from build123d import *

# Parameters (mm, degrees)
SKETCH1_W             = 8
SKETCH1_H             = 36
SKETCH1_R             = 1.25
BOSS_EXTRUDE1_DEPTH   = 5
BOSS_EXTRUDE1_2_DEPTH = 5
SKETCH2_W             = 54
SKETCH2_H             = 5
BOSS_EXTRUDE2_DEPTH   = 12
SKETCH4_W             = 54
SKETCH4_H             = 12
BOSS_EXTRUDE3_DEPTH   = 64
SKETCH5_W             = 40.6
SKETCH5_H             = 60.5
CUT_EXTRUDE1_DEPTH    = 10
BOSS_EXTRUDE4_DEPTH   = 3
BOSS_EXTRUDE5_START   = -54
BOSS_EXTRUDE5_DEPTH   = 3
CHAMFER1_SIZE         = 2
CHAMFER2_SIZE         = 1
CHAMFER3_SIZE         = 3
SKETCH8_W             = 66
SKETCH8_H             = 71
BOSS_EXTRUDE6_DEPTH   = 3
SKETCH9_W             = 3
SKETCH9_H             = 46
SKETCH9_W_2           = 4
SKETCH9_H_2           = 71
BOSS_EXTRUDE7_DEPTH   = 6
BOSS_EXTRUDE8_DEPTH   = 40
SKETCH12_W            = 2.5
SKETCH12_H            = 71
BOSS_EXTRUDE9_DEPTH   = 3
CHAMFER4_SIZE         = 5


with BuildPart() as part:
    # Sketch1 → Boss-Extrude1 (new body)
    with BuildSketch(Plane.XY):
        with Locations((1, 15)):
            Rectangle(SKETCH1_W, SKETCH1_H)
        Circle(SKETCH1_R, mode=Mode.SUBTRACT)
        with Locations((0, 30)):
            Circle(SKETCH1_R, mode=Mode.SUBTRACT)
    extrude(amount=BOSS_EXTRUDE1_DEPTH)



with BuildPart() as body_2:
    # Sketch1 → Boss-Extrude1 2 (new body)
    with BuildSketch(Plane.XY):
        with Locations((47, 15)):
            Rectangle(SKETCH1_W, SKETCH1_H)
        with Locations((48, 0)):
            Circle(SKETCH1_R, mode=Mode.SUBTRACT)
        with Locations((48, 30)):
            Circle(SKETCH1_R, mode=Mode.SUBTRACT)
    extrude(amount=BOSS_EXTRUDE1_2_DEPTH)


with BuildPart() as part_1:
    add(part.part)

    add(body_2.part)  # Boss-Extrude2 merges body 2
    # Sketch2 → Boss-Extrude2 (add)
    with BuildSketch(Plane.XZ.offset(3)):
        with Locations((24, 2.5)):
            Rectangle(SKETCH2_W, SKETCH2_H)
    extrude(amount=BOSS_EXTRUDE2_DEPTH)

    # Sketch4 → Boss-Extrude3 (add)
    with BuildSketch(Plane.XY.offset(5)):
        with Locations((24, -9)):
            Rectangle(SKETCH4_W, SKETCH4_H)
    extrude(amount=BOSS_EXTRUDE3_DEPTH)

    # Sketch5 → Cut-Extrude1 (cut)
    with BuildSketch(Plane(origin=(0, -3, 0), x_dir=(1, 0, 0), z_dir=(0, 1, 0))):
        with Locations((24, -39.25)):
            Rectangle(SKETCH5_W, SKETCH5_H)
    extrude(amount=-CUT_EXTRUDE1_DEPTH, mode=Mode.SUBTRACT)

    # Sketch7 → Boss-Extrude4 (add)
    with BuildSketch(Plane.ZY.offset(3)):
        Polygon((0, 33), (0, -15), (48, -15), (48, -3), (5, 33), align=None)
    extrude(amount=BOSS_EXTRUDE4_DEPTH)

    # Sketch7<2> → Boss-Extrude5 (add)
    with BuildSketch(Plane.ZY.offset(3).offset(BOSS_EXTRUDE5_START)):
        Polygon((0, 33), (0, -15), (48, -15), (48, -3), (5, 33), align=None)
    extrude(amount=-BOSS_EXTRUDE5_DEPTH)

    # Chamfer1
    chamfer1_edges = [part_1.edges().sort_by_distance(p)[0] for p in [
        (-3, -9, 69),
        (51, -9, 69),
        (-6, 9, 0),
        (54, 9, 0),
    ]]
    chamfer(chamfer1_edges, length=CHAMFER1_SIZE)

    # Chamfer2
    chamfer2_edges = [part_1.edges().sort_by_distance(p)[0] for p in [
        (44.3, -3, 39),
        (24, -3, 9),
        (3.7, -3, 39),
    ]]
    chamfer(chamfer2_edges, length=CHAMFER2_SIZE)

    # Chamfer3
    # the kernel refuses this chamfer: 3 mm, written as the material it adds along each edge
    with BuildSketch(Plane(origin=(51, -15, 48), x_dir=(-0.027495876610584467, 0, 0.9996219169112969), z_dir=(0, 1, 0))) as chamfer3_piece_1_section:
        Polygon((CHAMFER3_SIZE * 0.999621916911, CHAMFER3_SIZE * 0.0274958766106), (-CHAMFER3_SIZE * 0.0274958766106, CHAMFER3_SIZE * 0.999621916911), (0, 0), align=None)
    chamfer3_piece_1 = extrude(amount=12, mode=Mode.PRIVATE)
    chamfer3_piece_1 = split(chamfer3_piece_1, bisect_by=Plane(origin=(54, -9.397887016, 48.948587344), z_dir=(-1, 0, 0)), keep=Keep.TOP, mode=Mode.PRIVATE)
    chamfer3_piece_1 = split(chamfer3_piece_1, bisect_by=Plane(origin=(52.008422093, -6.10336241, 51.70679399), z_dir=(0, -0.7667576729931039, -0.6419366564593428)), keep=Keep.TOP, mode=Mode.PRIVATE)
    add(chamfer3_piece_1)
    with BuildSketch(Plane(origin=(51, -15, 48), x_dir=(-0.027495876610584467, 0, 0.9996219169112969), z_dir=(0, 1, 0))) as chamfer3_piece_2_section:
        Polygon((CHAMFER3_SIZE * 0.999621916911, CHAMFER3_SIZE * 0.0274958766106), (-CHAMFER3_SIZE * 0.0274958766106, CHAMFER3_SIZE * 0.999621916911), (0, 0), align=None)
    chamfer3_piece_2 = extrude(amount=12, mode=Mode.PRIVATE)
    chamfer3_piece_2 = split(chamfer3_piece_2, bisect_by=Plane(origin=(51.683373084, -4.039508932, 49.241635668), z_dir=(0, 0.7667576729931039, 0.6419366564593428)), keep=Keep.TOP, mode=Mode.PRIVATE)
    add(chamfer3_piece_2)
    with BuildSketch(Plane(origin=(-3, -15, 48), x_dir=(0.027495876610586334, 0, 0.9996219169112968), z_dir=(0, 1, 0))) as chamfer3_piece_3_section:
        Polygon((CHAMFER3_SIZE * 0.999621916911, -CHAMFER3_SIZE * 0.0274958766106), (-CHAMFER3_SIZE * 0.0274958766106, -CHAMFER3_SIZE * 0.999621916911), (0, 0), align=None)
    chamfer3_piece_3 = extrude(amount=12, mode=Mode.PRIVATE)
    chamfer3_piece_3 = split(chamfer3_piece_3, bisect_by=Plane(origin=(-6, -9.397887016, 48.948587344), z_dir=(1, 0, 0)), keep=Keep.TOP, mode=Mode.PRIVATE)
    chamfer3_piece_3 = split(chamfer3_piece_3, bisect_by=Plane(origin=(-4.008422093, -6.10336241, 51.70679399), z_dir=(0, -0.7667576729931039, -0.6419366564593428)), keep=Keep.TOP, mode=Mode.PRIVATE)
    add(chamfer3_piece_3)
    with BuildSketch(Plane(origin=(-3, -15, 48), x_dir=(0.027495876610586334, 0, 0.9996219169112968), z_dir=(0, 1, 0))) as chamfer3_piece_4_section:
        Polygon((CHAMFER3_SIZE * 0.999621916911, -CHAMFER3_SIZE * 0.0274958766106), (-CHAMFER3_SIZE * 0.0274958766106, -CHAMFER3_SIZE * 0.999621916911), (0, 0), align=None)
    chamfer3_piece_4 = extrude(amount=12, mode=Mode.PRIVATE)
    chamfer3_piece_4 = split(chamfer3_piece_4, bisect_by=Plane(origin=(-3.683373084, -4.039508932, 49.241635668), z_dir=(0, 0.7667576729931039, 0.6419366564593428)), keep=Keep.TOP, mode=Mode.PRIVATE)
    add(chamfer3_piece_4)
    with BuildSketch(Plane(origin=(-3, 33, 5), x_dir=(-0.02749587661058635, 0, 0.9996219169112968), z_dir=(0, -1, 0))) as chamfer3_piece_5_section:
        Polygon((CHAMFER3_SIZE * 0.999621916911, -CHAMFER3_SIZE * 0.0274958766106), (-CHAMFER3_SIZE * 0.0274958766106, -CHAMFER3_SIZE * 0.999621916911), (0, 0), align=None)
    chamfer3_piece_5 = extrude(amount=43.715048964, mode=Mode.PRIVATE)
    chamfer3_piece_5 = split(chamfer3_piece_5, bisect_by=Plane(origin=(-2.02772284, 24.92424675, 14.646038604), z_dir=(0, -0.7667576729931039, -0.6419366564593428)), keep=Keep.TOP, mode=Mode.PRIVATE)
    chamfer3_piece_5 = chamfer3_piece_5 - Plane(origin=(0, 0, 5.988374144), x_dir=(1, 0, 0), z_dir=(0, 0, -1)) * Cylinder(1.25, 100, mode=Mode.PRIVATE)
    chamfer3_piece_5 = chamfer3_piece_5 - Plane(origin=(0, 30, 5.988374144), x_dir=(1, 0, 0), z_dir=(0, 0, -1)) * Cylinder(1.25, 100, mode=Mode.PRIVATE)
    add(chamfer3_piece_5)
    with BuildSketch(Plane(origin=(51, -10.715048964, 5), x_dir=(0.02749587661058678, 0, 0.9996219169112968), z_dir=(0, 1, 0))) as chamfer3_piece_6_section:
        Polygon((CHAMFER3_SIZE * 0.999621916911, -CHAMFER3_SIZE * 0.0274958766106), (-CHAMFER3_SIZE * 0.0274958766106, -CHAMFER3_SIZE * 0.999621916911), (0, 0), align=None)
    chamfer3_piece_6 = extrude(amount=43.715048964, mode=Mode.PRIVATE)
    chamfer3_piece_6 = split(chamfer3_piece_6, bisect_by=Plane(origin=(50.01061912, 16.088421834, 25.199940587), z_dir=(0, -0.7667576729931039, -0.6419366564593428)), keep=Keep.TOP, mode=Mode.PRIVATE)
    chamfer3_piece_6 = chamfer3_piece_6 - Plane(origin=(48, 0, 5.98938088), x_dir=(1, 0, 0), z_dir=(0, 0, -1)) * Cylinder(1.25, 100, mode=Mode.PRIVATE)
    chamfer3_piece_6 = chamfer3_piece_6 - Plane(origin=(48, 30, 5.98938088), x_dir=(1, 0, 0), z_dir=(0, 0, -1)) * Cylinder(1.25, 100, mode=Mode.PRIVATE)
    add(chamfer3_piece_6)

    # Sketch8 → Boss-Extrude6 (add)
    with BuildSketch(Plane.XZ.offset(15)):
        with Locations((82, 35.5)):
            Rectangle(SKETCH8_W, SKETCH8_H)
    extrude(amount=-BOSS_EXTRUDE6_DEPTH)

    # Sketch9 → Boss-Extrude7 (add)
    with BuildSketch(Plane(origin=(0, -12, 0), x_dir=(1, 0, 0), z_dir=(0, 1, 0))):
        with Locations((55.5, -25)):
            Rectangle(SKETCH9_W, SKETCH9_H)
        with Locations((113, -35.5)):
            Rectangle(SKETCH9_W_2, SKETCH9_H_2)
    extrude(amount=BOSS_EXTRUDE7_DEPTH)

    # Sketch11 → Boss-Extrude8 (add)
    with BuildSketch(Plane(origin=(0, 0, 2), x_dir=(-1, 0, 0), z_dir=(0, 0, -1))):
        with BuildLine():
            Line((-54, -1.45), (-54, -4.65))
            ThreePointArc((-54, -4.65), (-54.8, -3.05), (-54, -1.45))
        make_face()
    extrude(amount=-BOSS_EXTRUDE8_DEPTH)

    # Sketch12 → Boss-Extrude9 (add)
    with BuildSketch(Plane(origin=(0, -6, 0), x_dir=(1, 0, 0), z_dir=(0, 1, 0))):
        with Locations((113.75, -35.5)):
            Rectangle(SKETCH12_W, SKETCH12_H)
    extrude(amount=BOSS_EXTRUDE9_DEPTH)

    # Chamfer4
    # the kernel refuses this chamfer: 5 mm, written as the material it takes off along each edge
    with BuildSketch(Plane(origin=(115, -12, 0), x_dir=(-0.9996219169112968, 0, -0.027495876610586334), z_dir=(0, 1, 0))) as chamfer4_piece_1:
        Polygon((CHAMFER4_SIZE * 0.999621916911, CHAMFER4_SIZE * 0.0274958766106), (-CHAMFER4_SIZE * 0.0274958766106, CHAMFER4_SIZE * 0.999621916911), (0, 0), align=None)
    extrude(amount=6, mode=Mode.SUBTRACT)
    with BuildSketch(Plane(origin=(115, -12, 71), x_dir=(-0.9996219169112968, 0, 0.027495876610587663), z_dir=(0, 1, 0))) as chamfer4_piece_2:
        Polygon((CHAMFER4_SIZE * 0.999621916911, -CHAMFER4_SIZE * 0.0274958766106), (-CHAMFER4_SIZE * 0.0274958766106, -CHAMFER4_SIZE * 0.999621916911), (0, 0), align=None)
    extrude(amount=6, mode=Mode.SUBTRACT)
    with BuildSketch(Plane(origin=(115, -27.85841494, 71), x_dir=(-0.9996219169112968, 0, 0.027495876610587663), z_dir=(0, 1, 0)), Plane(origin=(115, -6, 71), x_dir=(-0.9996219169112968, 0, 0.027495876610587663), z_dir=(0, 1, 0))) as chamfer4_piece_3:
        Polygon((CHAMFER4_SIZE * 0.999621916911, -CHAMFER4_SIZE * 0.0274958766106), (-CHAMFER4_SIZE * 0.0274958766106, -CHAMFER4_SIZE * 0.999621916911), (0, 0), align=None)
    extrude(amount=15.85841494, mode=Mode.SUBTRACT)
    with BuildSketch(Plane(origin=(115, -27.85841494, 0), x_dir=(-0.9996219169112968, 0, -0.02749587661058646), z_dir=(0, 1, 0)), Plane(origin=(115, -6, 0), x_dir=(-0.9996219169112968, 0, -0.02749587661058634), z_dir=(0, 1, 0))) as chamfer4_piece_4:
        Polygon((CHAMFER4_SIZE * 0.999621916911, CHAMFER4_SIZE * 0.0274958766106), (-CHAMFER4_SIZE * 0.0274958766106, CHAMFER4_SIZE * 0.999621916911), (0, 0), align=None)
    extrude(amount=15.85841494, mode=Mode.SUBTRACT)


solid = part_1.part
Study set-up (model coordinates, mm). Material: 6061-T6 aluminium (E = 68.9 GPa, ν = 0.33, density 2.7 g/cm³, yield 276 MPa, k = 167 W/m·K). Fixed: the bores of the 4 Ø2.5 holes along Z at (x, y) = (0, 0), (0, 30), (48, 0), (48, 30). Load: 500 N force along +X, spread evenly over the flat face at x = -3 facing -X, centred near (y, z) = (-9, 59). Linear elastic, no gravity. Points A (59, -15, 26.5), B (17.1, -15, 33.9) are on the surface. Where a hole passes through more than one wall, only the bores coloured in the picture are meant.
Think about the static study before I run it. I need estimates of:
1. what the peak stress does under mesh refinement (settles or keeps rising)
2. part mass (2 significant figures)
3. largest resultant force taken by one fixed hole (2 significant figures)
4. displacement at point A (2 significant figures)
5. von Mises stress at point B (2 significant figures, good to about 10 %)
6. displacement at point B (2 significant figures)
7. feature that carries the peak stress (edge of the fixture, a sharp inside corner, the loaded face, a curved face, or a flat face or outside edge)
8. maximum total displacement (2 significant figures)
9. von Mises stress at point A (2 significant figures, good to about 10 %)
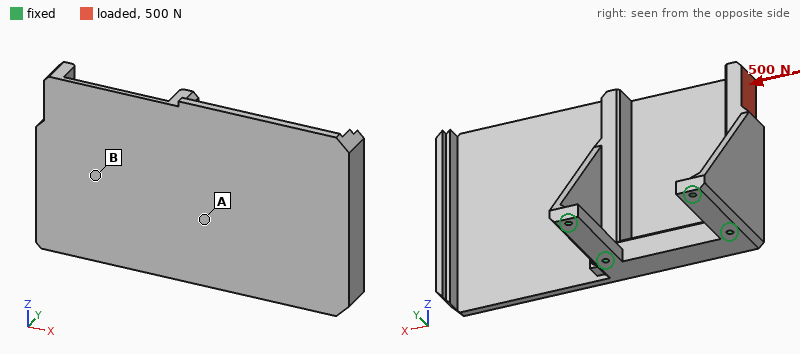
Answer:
keeps rising
130 g
800 N
18 µm
6.1 MPa
15 µm
edge of the fixture
66 µm
2.1 MPa
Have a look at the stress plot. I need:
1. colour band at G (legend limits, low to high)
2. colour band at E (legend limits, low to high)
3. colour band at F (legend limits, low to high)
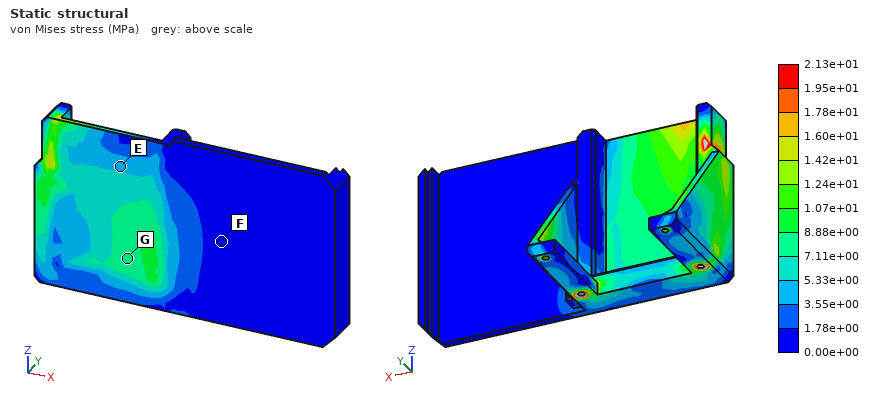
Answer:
7.11e+00 to 8.88e+00 MPa
3.55e+00 to 5.33e+00 MPa
0.00e+00 to 1.78e+00 MPa
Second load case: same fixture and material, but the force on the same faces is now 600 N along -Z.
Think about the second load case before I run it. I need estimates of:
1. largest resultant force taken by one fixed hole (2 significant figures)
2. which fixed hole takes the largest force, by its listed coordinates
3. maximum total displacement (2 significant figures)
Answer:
750 N
(0, 0)
26 µm
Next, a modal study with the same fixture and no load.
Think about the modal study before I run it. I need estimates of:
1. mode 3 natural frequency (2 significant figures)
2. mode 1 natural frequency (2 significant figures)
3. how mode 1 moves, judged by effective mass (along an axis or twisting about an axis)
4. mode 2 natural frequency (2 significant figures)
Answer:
2000 Hz
510 Hz
along Y
1200 Hz
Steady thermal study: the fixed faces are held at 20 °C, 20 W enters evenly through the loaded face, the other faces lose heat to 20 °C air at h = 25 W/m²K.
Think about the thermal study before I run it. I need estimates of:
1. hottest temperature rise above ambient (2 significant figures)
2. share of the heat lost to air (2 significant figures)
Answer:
35 K
21 %
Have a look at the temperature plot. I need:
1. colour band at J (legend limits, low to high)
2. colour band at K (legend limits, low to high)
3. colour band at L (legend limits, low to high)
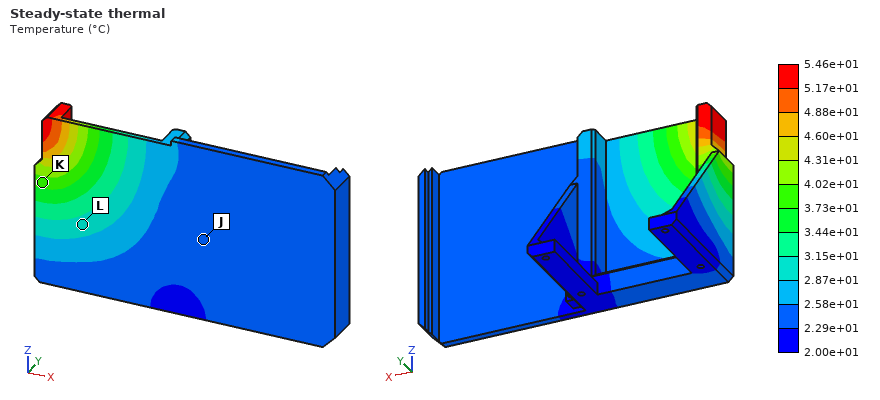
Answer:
2.29e+01 to 2.58e+01 °C
3.73e+01 to 4.02e+01 °C
2.87e+01 to 3.15e+01 °C
